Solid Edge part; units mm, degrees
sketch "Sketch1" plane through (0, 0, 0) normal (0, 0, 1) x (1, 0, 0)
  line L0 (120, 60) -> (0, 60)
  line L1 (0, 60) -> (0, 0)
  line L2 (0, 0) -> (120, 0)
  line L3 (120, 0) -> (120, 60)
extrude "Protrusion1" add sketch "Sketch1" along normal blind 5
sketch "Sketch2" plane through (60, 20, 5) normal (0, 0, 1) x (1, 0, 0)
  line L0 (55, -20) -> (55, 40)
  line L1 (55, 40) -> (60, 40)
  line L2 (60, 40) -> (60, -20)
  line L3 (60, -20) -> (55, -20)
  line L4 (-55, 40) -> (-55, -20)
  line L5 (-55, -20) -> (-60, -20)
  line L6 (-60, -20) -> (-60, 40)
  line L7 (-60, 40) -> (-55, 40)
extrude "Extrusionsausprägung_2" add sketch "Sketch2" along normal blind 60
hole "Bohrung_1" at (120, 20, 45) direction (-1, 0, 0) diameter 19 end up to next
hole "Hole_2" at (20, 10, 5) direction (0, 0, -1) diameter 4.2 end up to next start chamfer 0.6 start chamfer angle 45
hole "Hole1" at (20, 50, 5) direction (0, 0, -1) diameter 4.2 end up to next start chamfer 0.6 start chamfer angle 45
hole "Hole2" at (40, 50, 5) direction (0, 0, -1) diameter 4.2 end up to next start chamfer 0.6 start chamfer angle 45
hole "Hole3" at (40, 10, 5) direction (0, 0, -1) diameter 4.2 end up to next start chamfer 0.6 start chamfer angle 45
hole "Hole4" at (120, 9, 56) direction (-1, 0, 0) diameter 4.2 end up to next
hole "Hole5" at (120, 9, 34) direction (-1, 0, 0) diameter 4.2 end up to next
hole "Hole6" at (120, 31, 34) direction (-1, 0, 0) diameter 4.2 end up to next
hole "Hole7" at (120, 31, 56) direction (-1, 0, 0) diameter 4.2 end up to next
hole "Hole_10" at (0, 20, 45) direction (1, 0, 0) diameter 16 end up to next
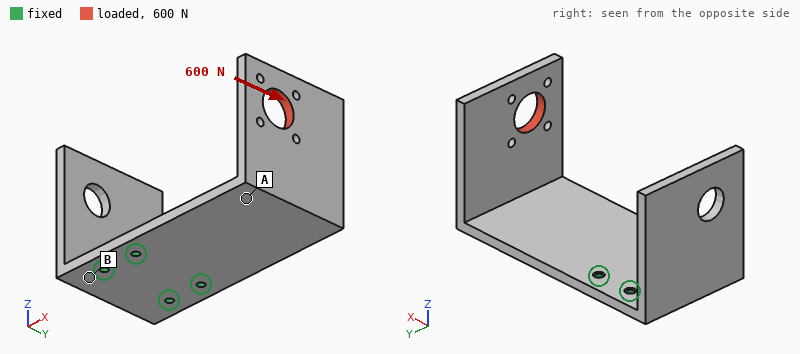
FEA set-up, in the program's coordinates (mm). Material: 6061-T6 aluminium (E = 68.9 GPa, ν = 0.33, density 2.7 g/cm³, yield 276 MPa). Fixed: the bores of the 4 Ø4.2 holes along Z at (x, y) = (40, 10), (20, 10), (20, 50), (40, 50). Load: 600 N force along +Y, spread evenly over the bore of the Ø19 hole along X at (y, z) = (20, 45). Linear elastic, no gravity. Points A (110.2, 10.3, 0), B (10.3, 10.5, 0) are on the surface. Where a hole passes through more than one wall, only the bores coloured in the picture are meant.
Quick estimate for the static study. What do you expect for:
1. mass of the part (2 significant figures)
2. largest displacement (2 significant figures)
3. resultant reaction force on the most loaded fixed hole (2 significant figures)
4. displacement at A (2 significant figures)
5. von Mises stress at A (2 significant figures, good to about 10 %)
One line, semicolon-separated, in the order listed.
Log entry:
190 g; 1.6 mm; 1.2 kN; 0.42 mm; 61 MPa
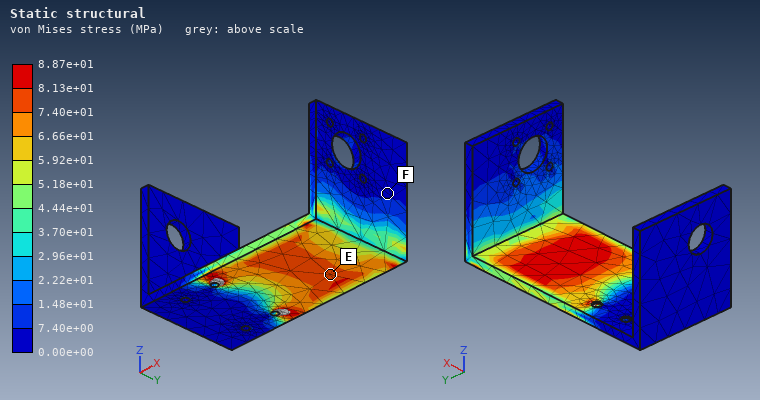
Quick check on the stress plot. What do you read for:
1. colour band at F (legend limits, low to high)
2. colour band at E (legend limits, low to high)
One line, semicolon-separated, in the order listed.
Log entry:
0.00e+00 to 7.40e+00 MPa; 7.40e+01 to 8.13e+01 MPa
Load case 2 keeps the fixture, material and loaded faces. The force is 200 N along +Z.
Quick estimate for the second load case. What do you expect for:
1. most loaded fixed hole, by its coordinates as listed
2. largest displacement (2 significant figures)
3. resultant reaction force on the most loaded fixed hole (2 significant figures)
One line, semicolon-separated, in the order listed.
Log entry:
(40, 10); 1.2 mm; 320 N
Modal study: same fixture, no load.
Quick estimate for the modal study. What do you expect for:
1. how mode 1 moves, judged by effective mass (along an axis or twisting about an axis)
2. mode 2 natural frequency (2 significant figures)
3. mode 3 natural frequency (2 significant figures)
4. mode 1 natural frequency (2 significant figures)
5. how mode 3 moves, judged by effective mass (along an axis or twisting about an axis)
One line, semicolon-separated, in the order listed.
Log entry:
along Z; 600 Hz; 760 Hz; 280 Hz; along X
